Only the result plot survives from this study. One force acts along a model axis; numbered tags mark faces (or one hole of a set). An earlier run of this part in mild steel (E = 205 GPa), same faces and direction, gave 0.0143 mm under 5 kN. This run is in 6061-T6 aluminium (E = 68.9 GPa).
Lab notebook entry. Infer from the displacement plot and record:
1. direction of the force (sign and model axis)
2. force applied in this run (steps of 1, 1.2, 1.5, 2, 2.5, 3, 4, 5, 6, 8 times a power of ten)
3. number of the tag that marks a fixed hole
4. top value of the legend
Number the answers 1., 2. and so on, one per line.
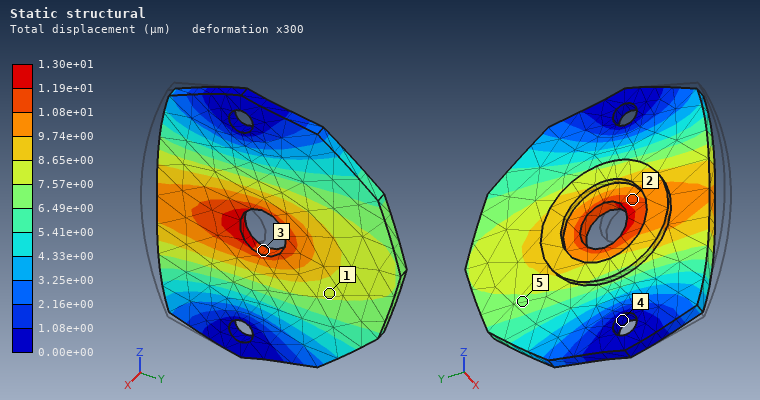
1. +Y
2. 1.5 kN
3. 4
4. 1.30e+01 µm
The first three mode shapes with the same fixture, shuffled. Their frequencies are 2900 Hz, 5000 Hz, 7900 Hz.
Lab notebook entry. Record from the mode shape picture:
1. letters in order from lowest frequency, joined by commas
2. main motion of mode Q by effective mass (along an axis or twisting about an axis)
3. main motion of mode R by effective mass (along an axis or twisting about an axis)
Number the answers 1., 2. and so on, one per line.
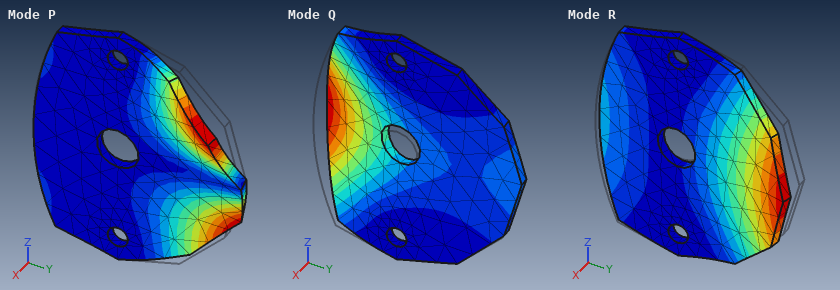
1. R, Q, P
2. along X
3. along X
